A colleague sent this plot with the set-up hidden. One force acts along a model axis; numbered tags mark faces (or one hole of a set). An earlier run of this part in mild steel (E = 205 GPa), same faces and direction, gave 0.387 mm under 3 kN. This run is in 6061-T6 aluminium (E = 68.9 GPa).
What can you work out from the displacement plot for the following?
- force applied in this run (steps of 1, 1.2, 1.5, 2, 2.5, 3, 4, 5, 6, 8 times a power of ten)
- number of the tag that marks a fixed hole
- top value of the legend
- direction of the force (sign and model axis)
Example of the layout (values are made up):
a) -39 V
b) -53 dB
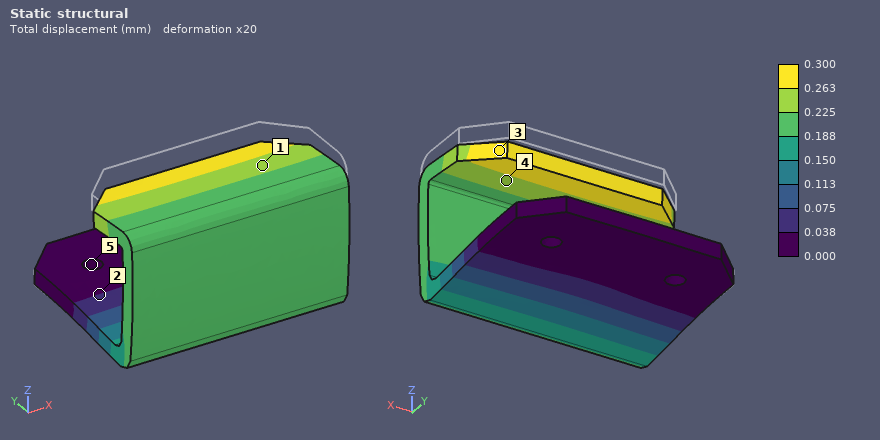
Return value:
a) 800 N
b) 5
c) 0.300 mm
d) -Z
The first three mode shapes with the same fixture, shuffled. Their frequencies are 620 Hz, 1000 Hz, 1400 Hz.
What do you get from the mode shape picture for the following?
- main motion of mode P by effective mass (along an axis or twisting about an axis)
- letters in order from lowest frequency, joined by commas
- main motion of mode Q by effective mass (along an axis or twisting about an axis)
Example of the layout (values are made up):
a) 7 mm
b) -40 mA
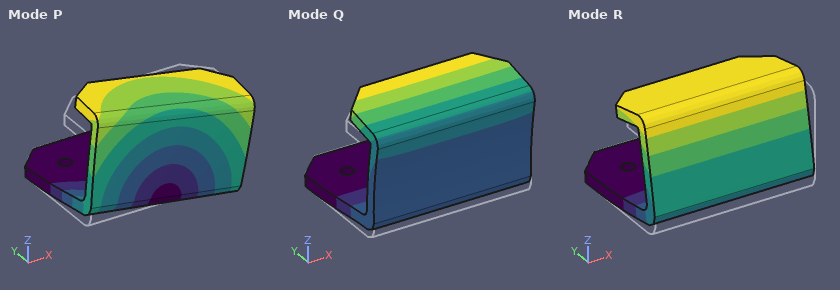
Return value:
a) along X
b) R, P, Q
c) along Z
